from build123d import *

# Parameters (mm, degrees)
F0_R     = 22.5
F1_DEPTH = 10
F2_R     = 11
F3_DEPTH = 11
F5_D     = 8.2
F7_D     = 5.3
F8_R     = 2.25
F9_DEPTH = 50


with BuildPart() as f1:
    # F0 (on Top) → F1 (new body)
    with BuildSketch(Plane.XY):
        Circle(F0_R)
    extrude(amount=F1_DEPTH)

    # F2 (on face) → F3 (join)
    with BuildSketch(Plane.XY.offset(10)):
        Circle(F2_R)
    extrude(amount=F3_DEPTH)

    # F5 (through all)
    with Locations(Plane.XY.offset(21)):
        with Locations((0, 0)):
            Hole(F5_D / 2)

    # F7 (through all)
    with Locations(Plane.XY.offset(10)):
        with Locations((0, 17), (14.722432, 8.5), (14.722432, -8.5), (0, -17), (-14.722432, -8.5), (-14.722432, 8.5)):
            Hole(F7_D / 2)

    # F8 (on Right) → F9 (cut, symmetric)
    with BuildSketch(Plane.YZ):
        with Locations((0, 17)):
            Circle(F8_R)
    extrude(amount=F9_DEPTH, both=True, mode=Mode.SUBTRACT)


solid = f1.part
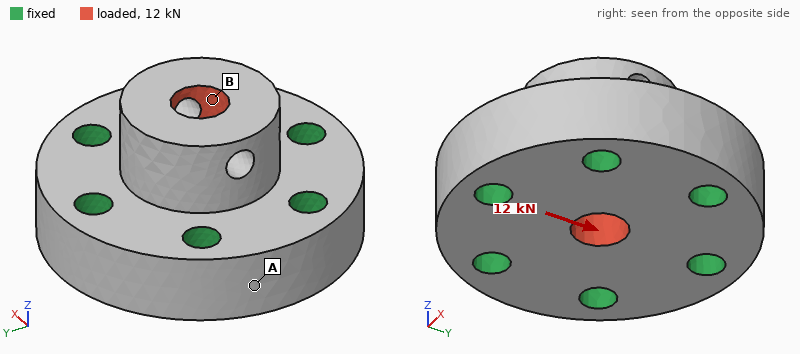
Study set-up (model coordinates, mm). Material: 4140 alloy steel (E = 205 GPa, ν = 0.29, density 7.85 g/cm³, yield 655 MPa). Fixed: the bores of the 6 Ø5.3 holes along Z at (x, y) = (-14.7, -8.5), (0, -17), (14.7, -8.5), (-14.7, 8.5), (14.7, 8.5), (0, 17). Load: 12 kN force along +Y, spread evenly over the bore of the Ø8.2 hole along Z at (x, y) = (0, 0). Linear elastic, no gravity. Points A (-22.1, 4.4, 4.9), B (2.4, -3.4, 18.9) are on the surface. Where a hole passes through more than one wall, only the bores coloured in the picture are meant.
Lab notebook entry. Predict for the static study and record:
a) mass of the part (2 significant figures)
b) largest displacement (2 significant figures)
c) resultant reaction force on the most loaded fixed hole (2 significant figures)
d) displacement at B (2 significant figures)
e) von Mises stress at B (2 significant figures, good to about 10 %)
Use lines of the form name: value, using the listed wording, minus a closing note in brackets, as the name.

mass of the part: 140 g
largest displacement: 6.1 µm
resultant reaction force on the most loaded fixed hole: 3.4 kN
displacement at B: 5.2 µm
von Mises stress at B: 30 MPa
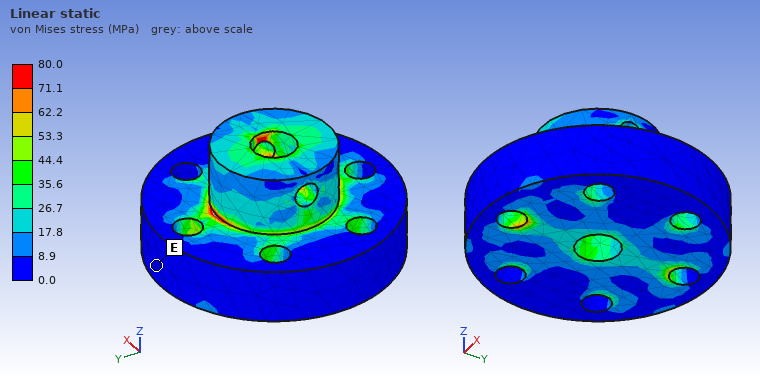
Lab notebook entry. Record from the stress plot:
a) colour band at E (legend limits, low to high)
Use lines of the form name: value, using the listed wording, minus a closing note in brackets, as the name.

colour band at E: 0.0 to 8.9 MPa
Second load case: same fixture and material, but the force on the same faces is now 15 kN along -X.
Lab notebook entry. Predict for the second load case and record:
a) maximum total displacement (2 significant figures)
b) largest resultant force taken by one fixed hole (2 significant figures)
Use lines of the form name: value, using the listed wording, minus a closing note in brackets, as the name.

maximum total displacement: 6.8 µm
largest resultant force taken by one fixed hole: 3.7 kN
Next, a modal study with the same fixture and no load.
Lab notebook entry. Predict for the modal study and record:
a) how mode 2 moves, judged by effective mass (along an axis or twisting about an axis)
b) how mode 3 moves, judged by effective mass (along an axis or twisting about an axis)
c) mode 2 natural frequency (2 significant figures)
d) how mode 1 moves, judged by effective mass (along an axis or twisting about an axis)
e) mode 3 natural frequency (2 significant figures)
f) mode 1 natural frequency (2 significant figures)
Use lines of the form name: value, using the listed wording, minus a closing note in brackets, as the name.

how mode 2 moves, judged by effective mass: along X
how mode 3 moves, judged by effective mass: along Z
mode 2 natural frequency: 40 kHz
how mode 1 moves, judged by effective mass: along Y
mode 3 natural frequency: 47 kHz
mode 1 natural frequency: 38 kHz
